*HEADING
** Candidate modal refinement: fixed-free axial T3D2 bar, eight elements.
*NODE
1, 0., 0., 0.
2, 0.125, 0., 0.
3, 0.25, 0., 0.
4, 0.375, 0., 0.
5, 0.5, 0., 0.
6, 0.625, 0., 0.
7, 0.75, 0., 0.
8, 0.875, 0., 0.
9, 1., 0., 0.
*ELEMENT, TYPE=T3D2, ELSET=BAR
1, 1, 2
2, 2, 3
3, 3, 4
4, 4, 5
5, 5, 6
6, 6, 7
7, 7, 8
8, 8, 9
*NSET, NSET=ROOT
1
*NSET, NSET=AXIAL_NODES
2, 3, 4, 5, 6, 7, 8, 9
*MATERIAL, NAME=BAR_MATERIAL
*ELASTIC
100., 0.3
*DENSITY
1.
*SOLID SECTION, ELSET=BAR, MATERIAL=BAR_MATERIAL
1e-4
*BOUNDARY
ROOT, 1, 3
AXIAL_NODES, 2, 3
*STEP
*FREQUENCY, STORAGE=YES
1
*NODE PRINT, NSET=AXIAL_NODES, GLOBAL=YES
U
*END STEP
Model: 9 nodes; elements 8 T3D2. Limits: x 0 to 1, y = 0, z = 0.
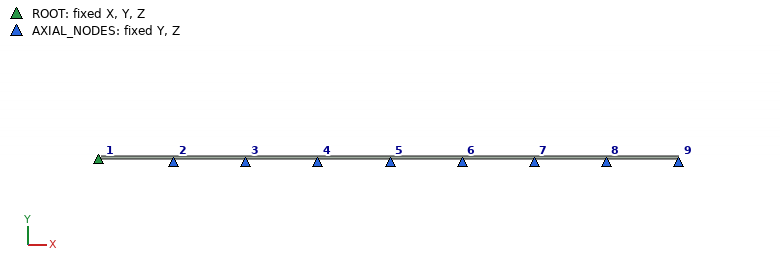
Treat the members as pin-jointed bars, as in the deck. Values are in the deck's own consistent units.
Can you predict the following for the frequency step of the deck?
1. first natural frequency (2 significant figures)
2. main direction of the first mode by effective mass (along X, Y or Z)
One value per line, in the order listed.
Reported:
2.5 cycles per unit time
along X
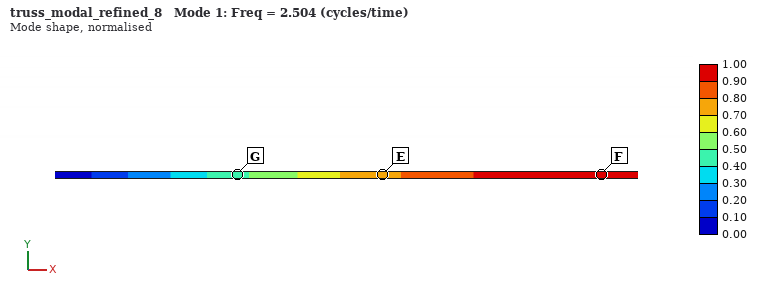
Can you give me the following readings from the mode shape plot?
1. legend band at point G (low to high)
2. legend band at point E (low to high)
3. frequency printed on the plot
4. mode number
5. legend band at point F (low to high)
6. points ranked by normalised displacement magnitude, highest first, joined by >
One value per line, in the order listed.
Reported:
0.40 to 0.50
0.70 to 0.80
2.504
1
0.90 to 1.00
F > E > G
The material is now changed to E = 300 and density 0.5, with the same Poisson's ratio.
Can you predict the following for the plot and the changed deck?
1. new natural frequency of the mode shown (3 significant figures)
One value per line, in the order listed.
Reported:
6.13
